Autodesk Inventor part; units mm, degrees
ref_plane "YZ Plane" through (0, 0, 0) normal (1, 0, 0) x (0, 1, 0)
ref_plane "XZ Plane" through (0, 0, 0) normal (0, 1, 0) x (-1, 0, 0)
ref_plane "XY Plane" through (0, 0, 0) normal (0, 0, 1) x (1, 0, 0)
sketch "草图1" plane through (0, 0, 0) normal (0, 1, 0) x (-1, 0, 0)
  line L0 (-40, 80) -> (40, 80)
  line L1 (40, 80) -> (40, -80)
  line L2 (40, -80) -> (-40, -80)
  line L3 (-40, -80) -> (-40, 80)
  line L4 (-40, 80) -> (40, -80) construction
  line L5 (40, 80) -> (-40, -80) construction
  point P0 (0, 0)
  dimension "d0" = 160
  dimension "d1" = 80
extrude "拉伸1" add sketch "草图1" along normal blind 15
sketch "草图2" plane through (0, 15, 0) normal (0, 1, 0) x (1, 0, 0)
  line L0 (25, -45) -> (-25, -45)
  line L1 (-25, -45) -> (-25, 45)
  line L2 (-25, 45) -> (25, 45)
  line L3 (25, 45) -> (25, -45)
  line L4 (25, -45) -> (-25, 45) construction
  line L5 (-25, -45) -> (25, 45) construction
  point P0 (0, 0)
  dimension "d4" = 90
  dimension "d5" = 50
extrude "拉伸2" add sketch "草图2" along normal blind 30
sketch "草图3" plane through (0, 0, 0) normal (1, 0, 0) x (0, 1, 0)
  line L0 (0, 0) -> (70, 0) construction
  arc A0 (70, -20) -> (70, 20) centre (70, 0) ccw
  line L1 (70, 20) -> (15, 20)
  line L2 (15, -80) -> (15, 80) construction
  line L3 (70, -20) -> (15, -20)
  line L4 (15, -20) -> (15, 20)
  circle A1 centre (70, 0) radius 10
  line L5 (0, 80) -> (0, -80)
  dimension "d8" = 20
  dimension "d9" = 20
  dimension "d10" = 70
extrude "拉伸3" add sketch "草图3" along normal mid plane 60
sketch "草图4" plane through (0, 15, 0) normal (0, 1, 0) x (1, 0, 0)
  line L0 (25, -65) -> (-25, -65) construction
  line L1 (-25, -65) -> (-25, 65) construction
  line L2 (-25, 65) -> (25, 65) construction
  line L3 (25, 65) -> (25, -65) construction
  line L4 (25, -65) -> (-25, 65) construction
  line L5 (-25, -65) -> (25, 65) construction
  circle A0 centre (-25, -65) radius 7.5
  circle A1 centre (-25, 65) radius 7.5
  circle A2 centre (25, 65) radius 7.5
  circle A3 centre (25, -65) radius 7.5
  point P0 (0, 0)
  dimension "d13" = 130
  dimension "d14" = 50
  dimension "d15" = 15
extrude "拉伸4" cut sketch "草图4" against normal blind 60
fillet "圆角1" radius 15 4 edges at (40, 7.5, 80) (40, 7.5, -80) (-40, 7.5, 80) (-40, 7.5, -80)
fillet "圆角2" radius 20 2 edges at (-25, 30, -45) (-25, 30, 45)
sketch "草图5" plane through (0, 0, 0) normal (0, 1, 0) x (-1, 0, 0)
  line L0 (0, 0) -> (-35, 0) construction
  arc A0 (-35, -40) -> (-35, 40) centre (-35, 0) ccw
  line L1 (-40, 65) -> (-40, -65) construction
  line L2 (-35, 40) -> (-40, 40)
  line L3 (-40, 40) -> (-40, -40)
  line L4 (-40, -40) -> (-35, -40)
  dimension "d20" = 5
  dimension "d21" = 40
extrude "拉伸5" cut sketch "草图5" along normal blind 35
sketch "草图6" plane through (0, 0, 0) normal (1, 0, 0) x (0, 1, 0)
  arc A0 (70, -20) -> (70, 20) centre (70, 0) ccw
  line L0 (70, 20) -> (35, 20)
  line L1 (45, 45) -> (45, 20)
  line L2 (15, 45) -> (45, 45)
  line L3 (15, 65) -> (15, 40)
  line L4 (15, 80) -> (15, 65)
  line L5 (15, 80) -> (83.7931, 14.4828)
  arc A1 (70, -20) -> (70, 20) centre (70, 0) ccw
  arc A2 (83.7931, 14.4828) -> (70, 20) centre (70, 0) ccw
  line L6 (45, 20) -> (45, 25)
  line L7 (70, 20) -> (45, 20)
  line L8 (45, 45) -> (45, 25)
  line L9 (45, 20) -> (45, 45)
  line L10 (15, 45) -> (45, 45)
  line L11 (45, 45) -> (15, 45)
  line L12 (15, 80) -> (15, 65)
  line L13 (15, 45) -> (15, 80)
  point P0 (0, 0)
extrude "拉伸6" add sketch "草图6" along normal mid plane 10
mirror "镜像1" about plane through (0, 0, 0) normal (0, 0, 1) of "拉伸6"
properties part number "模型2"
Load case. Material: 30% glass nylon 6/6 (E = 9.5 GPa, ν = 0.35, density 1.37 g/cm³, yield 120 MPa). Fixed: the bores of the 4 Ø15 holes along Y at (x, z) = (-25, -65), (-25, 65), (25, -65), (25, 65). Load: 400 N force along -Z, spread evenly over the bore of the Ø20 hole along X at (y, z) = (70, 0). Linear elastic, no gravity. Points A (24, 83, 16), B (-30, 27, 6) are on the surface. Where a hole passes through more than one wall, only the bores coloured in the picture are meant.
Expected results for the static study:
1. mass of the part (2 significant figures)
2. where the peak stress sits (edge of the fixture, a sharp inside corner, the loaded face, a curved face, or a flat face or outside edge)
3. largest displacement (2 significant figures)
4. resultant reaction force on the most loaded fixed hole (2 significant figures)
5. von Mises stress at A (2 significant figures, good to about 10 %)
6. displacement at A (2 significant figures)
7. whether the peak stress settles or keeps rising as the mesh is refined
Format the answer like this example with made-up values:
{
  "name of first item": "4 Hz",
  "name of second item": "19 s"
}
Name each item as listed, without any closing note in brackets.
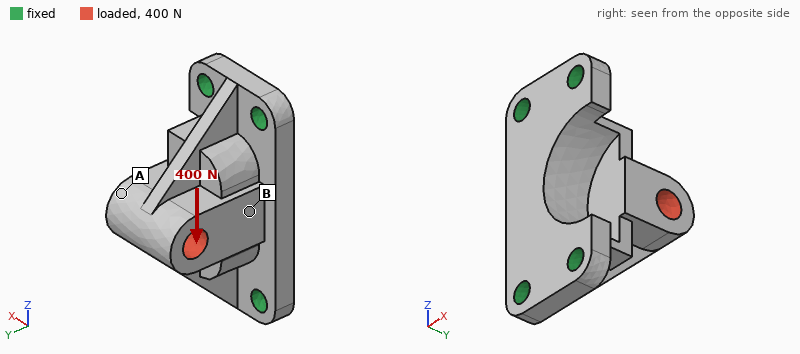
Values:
{
  "mass of the part": "470 g",
  "where the peak stress sits": "edge of the fixture",
  "largest displacement": "10 µm",
  "resultant reaction force on the most loaded fixed hole": "170 N",
  "von Mises stress at A": "0.25 MPa",
  "displacement at A": "9.6 µm",
  "whether the peak stress settles or keeps rising as the mesh is refined": "keeps rising"
}
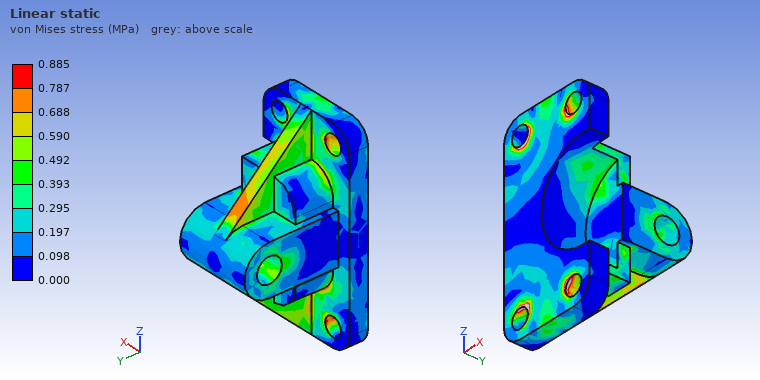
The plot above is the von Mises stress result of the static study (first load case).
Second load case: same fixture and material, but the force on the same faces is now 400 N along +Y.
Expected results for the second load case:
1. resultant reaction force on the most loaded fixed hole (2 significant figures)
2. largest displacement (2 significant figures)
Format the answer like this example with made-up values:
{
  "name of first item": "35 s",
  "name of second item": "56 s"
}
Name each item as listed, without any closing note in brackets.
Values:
{
  "resultant reaction force on the most loaded fixed hole": "120 N",
  "largest displacement": "8.2 µm"
}
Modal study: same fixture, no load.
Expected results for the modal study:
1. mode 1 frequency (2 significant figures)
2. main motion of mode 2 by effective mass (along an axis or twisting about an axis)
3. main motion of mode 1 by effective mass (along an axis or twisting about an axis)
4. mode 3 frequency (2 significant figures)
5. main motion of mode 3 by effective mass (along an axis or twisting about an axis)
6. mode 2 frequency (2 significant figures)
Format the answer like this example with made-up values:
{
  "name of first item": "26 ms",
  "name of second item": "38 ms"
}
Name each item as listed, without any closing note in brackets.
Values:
{
  "mode 1 frequency": "1300 Hz",
  "main motion of mode 2 by effective mass": "along Y",
  "main motion of mode 1 by effective mass": "along X",
  "mode 3 frequency": "3200 Hz",
  "main motion of mode 3 by effective mass": "along Z",
  "mode 2 frequency": "2800 Hz"
}
